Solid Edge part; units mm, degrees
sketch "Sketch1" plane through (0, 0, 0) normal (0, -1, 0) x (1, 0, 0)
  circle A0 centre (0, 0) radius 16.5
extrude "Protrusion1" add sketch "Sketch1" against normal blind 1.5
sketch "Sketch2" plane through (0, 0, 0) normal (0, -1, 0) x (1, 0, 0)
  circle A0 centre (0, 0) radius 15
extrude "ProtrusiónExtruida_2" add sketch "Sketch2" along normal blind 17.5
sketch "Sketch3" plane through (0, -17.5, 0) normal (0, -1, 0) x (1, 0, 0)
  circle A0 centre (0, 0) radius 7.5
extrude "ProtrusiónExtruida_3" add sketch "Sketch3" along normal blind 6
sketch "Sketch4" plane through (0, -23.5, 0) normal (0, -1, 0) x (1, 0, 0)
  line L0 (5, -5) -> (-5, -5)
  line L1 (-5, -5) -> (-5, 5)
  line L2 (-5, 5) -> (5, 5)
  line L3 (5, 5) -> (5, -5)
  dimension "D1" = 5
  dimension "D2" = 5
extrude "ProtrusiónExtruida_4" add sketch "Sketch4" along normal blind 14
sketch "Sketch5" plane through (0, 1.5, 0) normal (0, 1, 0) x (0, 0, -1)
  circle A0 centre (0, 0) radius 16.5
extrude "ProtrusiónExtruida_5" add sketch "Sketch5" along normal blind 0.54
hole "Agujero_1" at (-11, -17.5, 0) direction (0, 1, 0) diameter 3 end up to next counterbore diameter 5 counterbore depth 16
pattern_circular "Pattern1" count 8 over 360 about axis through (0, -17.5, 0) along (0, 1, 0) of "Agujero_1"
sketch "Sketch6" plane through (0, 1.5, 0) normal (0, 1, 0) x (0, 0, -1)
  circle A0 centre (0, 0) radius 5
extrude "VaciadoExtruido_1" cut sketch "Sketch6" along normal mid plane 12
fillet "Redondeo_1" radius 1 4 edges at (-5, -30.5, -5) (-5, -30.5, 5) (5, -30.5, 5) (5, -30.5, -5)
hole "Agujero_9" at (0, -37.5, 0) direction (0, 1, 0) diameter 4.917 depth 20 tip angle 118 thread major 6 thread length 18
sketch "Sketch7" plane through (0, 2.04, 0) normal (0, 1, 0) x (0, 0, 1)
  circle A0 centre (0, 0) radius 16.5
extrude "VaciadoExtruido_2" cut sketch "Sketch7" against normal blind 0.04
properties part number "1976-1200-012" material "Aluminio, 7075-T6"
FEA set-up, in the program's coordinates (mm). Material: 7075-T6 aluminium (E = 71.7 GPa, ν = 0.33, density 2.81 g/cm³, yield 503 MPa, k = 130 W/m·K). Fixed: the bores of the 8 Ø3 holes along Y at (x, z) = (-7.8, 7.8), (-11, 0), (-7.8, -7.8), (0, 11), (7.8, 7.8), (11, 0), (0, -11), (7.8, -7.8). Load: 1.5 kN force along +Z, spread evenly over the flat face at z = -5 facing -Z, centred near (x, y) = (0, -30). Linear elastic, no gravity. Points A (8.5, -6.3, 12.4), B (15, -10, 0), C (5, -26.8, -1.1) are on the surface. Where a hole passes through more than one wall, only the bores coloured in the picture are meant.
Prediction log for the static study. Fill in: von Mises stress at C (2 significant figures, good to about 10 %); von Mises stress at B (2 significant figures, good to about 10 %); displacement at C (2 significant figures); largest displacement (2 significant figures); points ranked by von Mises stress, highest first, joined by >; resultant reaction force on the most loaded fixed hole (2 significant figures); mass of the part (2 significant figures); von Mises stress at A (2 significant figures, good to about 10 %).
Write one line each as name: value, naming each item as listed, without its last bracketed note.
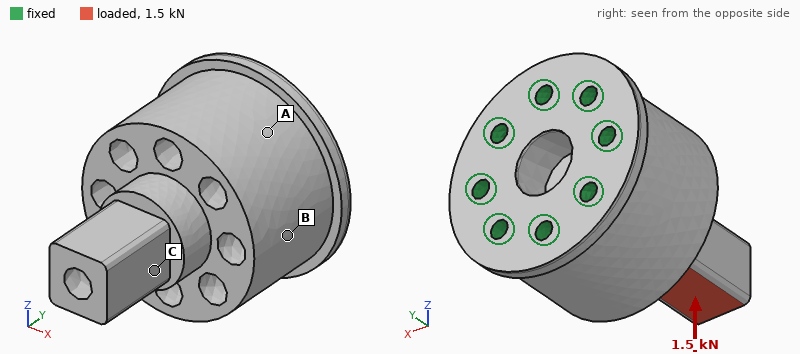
von Mises stress at C: 43 MPa
von Mises stress at B: 6.1 MPa
displacement at C: 25 µm
largest displacement: 58 µm
points ranked by von Mises stress, highest first, joined by >: C > A > B
resultant reaction force on the most loaded fixed hole: 1000 N
mass of the part: 36 g
von Mises stress at A: 12 MPa
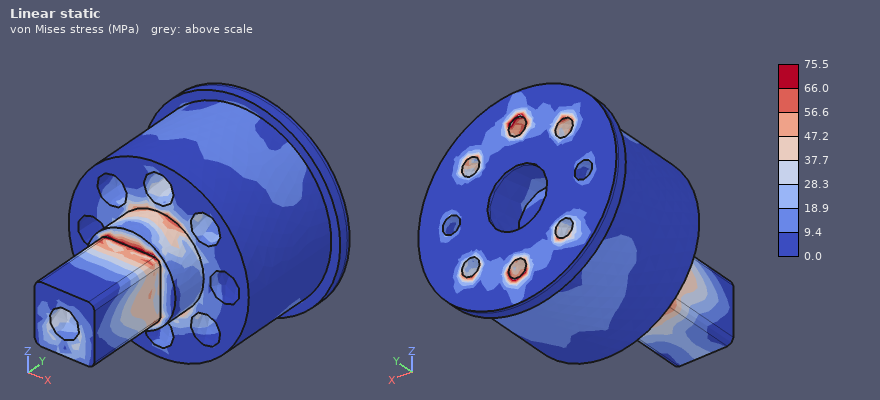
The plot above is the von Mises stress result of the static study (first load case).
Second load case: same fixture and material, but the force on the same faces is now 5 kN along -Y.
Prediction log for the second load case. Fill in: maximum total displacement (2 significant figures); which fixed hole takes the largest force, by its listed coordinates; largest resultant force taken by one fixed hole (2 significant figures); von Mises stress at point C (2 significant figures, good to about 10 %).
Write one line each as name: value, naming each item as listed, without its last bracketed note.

maximum total displacement: 88 µm
which fixed hole takes the largest force, by its listed coordinates: (0, -11)
largest resultant force taken by one fixed hole: 1.2 kN
von Mises stress at point C: 60 MPa
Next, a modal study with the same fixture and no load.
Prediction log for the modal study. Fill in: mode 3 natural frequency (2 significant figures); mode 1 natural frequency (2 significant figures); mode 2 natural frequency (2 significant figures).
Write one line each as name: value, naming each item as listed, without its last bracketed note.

mode 3 natural frequency: 29 kHz
mode 1 natural frequency: 15 kHz
mode 2 natural frequency: 15 kHz
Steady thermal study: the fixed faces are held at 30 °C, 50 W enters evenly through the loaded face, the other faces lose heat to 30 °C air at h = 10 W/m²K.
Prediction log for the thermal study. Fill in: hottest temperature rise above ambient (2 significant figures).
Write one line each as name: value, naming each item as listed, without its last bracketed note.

hottest temperature rise above ambient: 84 K
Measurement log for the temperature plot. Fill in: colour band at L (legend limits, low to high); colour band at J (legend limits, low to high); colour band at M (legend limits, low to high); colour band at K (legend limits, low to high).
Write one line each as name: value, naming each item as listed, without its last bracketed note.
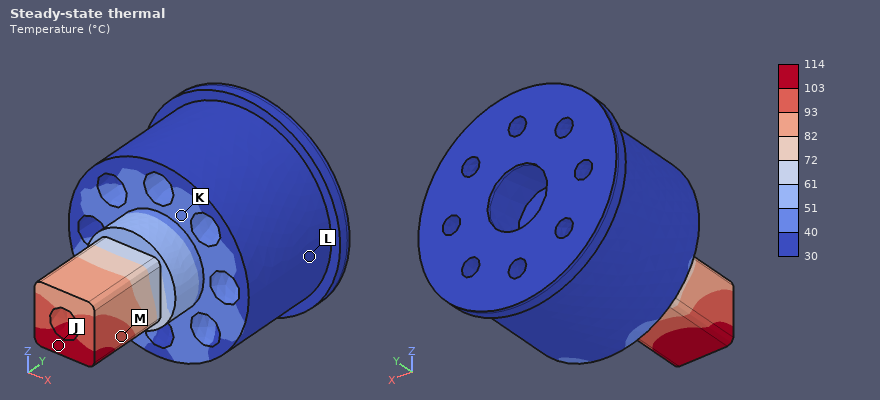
colour band at L: 30 to 40 °C
colour band at J: 103 to 114 °C
colour band at M: 93 to 103 °C
colour band at K: 40 to 51 °C
